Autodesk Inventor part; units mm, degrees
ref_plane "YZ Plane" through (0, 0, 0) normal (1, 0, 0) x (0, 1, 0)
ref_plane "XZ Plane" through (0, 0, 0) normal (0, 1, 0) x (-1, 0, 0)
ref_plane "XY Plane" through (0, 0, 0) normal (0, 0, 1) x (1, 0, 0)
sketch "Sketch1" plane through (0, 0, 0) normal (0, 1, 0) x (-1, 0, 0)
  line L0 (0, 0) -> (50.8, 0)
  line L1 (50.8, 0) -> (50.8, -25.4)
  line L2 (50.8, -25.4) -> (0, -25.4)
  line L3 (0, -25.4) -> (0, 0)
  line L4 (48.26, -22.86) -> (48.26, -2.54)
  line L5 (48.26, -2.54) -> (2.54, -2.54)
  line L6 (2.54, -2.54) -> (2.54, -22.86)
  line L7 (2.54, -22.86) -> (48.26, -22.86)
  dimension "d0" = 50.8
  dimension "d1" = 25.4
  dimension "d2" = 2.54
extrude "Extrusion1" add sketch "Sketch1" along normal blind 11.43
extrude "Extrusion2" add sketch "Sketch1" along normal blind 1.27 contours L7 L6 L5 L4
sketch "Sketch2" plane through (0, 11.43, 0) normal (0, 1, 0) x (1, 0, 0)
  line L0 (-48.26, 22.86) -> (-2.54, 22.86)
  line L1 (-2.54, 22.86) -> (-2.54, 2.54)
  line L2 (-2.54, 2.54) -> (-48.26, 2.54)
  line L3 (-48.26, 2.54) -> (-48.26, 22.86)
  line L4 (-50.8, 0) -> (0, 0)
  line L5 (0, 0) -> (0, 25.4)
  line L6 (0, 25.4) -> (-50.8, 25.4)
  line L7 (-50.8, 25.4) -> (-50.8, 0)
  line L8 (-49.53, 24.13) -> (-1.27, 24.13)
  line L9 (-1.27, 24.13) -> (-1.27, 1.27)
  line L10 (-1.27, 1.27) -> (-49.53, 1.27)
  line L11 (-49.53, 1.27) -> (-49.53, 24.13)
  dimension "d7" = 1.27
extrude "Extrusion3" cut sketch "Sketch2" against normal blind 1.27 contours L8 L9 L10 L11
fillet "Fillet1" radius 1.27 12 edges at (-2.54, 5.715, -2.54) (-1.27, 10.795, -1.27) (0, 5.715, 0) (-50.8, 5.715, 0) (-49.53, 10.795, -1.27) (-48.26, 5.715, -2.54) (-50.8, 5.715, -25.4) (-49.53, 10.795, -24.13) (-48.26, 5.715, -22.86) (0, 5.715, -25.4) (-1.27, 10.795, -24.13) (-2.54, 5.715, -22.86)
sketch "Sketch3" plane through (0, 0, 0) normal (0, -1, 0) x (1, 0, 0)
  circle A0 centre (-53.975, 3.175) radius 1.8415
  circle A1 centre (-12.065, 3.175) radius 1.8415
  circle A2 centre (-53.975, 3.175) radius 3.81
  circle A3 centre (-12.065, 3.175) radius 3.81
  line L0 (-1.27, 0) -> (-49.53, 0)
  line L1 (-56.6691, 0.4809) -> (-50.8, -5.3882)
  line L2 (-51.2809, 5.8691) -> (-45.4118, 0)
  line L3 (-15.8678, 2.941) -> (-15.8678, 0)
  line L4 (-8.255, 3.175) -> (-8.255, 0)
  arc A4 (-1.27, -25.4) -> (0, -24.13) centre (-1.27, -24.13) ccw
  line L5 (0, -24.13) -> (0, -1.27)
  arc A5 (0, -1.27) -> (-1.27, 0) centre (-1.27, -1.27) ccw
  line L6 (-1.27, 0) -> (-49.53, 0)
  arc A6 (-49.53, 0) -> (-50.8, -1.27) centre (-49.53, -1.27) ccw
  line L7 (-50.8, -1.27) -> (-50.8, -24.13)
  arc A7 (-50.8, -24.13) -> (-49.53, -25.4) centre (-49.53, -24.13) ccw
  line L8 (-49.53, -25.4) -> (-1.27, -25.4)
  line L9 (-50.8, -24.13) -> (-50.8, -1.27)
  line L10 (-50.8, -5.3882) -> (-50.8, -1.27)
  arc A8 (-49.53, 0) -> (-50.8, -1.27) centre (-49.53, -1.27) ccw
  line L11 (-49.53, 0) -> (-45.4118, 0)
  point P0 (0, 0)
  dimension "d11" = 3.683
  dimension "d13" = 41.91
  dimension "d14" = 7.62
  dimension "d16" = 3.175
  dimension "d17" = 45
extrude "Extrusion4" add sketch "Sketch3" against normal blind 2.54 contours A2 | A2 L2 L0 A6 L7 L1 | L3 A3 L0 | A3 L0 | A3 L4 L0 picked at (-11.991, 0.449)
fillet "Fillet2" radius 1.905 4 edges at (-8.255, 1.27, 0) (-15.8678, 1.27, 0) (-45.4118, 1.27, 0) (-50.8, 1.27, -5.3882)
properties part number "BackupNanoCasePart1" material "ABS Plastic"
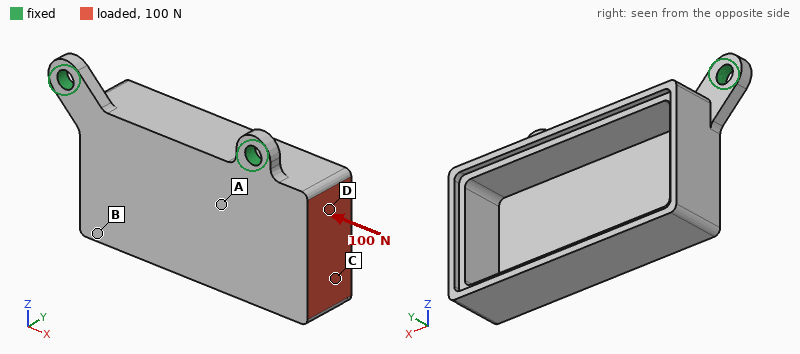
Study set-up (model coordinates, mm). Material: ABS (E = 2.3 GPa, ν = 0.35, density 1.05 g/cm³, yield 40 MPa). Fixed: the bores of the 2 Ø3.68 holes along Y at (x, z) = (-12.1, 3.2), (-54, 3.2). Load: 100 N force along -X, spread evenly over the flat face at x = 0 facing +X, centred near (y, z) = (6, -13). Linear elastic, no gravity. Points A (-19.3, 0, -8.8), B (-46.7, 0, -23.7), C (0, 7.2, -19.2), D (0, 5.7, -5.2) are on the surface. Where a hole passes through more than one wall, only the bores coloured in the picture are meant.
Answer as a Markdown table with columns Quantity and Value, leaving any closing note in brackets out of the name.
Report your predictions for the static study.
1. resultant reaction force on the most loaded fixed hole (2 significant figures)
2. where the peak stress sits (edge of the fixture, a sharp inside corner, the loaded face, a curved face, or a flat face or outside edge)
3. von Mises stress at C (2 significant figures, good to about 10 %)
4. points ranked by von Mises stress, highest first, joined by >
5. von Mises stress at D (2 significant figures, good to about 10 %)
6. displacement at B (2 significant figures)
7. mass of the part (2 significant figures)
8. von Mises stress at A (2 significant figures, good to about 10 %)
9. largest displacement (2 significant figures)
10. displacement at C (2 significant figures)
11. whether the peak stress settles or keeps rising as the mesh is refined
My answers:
| Quantity | Value |
|---|---|
| resultant reaction force on the most loaded fixed hole | 61 N |
| where the peak stress sits | edge of the fixture |
| von Mises stress at C | 5.0 MPa |
| points ranked by von Mises stress, highest first, joined by > | D > C > A > B |
| von Mises stress at D | 7.1 MPa |
| displacement at B | 0.31 mm |
| mass of the part | 5.6 g |
| von Mises stress at A | 2.3 MPa |
| largest displacement | 0.43 mm |
| displacement at C | 0.33 mm |
| whether the peak stress settles or keeps rising as the mesh is refined | keeps rising |
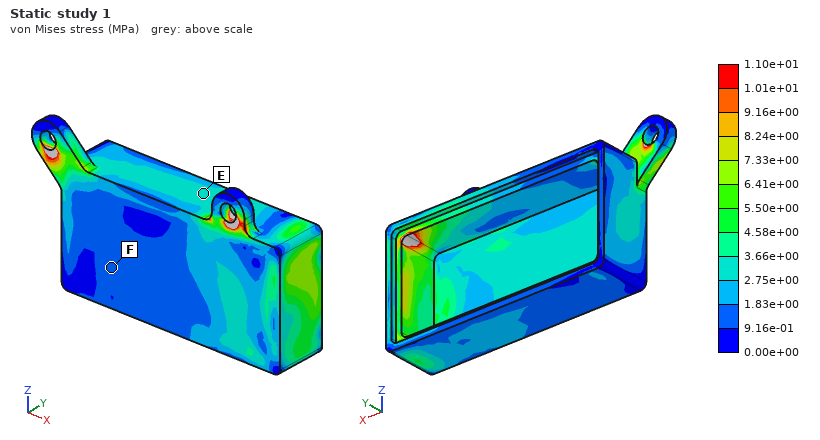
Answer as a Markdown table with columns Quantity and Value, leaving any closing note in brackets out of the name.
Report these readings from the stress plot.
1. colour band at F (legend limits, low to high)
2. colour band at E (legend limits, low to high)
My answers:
| Quantity | Value |
|---|---|
| colour band at F | 9.16e-01 to 1.83e+00 MPa |
| colour band at E | 2.75e+00 to 3.66e+00 MPa |
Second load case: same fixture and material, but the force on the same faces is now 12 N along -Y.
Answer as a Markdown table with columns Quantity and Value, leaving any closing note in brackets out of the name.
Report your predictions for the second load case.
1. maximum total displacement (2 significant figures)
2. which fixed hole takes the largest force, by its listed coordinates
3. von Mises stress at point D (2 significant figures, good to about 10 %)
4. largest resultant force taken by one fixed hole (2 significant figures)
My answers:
| Quantity | Value |
|---|---|
| maximum total displacement | 0.68 mm |
| which fixed hole takes the largest force, by its listed coordinates | (-12.1, 3.2) |
| von Mises stress at point D | 1.6 MPa |
| largest resultant force taken by one fixed hole | 16 N |
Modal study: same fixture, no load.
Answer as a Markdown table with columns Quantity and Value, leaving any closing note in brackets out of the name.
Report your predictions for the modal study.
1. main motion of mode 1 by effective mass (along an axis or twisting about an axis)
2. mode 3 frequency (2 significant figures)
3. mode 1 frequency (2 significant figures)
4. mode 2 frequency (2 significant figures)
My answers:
| Quantity | Value |
|---|---|
| main motion of mode 1 by effective mass | along Y |
| mode 3 frequency | 2500 Hz |
| mode 1 frequency | 410 Hz |
| mode 2 frequency | 860 Hz |
